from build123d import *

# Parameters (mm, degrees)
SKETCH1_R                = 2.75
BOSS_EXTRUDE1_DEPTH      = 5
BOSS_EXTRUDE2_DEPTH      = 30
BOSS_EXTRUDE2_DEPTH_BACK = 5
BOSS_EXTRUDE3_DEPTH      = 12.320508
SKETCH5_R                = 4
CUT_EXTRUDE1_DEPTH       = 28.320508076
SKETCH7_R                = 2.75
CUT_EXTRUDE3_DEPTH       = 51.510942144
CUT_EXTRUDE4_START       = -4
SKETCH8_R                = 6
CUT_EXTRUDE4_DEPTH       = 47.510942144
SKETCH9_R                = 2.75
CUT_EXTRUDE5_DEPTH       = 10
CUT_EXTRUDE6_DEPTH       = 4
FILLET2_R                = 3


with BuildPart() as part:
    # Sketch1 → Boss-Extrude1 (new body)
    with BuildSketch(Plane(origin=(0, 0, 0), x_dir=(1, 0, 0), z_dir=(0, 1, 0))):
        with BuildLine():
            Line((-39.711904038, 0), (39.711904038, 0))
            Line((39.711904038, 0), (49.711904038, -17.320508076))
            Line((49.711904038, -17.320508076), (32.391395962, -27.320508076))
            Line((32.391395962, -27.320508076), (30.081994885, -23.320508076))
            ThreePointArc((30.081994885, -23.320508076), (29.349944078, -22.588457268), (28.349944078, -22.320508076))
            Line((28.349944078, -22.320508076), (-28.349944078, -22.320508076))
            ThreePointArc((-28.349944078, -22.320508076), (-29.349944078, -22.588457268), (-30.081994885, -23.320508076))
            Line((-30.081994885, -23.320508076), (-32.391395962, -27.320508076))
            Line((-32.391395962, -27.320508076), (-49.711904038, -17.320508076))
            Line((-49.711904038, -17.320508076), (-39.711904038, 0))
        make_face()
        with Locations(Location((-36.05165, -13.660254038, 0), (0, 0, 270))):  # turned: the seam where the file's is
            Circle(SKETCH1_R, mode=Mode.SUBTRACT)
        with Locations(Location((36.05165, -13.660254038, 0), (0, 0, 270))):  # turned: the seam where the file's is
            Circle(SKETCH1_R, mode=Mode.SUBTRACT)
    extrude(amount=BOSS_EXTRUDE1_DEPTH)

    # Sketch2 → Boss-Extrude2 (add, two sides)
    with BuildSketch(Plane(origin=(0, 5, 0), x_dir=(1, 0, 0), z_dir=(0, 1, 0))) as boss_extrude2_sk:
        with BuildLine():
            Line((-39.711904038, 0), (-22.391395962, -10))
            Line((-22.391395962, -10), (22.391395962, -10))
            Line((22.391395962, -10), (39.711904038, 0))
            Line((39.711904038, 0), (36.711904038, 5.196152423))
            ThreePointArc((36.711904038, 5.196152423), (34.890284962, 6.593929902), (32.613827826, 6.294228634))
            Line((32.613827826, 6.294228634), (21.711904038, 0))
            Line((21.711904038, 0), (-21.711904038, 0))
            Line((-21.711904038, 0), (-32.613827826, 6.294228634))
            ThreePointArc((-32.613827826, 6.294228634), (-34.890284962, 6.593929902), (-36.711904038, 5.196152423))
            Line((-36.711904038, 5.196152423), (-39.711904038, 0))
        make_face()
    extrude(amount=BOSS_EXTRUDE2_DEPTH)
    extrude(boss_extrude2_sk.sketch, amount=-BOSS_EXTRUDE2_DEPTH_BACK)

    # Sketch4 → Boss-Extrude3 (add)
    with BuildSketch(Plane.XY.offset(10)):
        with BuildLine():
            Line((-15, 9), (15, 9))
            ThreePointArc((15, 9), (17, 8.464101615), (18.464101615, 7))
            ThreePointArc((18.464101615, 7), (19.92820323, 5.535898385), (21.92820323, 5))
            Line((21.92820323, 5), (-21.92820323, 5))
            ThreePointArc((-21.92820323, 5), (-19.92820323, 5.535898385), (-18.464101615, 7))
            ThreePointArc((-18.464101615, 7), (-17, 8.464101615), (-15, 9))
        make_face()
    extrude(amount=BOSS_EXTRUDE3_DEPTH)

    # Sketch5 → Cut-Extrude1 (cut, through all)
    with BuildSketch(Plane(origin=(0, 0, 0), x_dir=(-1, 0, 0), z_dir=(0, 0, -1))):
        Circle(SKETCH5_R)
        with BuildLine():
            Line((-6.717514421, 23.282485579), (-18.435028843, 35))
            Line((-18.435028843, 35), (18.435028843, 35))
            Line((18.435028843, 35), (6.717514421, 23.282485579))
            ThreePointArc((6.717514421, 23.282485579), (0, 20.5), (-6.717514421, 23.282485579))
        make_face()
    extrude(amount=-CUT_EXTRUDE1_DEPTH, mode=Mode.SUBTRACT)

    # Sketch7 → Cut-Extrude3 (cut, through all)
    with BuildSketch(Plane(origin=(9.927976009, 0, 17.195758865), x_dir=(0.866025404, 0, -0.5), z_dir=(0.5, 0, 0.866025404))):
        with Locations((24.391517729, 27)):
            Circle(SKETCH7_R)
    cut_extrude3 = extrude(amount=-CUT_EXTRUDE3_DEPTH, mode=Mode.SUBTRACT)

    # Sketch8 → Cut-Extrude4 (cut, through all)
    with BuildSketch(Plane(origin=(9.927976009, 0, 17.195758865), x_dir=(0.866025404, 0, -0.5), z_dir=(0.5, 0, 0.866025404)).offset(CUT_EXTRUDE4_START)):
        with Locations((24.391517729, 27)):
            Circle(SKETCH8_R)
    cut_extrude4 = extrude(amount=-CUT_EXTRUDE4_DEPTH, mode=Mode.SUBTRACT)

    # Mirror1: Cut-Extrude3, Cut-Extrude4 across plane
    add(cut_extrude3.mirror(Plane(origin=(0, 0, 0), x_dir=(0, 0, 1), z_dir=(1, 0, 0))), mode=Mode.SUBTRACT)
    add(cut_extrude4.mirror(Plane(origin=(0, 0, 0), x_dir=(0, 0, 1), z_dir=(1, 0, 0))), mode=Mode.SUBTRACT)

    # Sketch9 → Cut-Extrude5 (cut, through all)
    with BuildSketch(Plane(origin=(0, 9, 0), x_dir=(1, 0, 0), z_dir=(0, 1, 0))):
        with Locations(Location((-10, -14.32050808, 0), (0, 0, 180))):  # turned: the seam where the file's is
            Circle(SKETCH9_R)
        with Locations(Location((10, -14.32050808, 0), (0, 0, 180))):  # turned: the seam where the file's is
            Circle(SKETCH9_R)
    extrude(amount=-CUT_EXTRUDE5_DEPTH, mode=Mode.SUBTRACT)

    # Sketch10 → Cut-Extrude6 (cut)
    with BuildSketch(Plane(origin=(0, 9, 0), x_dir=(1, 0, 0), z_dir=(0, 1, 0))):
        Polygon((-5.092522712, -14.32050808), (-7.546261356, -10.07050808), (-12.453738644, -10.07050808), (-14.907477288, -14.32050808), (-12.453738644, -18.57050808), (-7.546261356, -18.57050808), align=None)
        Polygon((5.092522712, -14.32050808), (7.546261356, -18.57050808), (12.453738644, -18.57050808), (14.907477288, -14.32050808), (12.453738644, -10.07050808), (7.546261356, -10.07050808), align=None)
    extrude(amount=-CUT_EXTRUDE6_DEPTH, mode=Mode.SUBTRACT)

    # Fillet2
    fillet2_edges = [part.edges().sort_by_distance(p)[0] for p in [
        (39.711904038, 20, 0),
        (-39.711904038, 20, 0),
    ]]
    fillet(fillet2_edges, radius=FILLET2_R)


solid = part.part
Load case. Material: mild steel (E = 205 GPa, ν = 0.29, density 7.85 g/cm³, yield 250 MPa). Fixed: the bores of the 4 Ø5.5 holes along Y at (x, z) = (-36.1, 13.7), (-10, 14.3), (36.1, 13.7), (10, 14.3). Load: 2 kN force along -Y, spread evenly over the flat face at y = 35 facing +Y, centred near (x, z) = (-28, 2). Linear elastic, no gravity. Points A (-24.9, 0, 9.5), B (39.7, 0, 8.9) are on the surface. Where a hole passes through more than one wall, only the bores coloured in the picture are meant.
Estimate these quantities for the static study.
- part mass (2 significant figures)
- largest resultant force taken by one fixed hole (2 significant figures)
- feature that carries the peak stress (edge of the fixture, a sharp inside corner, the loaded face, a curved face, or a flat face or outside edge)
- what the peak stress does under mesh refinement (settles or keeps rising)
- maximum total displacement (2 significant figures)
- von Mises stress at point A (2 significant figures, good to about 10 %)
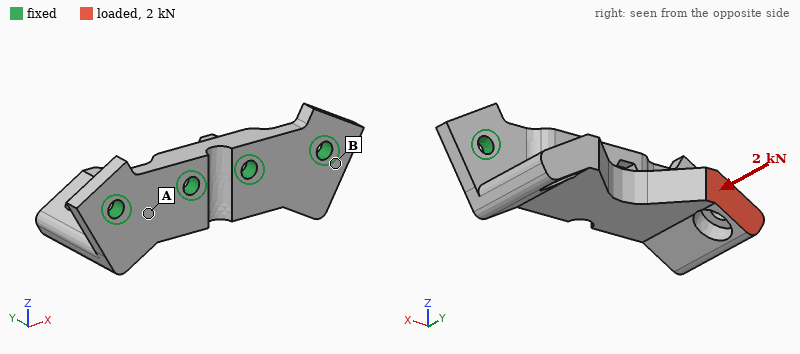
230 g
1.1 kN
edge of the fixture
keeps rising
31 µm
29 MPa
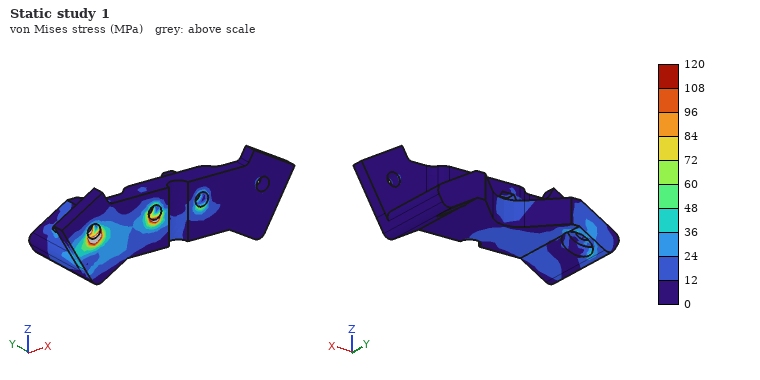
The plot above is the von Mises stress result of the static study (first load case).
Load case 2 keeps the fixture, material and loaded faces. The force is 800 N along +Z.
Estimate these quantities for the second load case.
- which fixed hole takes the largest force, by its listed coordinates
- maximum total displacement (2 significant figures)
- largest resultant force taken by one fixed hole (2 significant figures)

(-10, 14.3)
54 µm
640 N
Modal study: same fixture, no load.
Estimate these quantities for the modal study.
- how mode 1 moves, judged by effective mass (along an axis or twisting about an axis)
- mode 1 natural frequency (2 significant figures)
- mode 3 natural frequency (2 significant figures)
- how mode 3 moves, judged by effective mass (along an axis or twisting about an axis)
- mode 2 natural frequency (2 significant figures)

along Z
4100 Hz
11 kHz
along X
5900 Hz
